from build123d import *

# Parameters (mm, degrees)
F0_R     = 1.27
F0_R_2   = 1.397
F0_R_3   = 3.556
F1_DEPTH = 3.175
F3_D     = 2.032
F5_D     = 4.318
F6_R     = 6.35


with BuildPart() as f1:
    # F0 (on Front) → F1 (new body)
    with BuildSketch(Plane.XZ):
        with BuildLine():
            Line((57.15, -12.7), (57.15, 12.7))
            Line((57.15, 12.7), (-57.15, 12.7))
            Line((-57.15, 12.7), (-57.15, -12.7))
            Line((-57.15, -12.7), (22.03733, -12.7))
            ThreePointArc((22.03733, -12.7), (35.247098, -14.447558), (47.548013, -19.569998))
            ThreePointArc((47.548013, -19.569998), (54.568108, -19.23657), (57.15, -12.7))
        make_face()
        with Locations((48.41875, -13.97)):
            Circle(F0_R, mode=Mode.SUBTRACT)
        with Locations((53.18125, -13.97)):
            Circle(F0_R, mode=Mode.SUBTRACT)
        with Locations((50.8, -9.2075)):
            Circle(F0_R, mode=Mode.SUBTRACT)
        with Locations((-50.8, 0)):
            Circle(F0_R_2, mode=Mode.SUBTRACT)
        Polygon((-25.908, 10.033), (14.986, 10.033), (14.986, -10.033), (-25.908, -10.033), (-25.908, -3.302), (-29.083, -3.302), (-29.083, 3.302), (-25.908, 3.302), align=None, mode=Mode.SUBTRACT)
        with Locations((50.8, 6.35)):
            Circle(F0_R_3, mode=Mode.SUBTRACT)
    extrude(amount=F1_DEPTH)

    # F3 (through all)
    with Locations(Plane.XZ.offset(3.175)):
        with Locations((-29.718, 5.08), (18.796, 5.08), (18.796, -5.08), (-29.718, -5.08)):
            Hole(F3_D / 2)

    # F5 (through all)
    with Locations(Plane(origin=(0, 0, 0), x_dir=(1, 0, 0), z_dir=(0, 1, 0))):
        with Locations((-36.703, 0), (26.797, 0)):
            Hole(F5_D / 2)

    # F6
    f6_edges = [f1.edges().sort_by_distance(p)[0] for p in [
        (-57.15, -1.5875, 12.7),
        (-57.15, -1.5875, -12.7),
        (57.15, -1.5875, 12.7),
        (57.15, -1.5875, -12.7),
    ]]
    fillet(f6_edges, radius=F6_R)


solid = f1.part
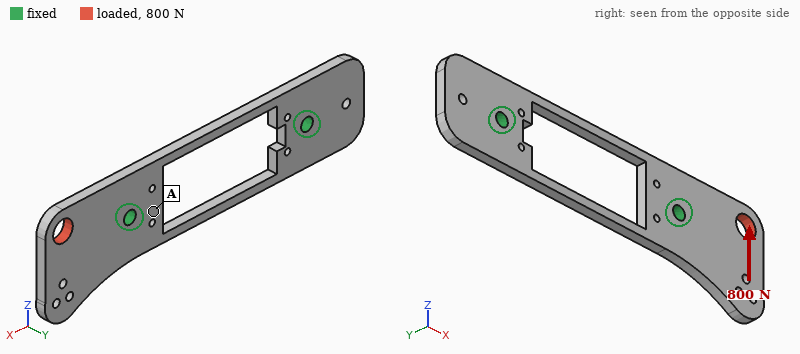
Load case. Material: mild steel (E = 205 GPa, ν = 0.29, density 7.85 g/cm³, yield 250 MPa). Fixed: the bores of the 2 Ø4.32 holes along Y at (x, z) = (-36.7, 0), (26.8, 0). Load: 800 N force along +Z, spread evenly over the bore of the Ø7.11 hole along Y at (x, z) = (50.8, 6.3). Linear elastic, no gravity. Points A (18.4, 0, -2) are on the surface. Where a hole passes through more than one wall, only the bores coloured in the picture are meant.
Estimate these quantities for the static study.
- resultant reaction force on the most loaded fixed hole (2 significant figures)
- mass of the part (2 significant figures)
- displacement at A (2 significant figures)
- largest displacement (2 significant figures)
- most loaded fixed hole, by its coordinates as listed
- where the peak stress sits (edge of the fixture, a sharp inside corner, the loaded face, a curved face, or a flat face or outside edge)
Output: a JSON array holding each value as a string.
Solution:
["810 N", "51 g", "6.7 µm", "39 µm", "(26.8, 0)", "edge of the fixture"]
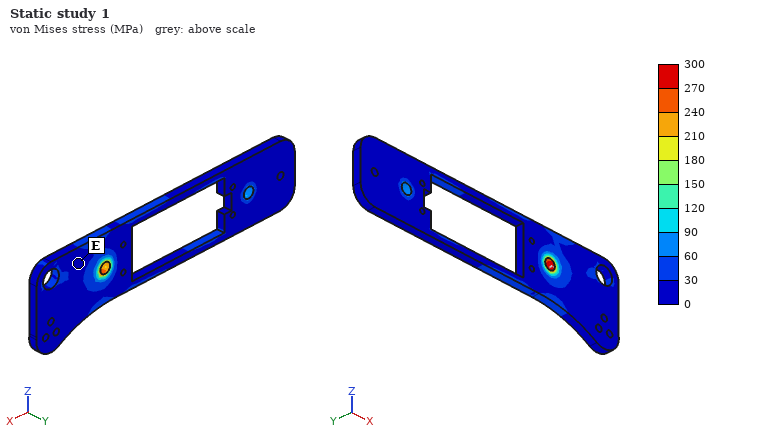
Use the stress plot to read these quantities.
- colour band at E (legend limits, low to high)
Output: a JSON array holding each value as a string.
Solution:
["0 to 30 MPa"]
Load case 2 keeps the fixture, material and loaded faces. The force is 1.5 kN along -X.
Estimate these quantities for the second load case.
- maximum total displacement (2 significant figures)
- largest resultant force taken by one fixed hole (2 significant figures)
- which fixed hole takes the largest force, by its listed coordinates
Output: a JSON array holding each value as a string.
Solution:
["21 µm", "1.4 kN", "(26.8, 0)"]
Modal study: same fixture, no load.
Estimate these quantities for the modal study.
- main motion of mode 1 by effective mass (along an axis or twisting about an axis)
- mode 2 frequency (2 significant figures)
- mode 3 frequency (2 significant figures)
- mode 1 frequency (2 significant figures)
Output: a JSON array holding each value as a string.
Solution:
["along Y", "5200 Hz", "5400 Hz", "2700 Hz"]
